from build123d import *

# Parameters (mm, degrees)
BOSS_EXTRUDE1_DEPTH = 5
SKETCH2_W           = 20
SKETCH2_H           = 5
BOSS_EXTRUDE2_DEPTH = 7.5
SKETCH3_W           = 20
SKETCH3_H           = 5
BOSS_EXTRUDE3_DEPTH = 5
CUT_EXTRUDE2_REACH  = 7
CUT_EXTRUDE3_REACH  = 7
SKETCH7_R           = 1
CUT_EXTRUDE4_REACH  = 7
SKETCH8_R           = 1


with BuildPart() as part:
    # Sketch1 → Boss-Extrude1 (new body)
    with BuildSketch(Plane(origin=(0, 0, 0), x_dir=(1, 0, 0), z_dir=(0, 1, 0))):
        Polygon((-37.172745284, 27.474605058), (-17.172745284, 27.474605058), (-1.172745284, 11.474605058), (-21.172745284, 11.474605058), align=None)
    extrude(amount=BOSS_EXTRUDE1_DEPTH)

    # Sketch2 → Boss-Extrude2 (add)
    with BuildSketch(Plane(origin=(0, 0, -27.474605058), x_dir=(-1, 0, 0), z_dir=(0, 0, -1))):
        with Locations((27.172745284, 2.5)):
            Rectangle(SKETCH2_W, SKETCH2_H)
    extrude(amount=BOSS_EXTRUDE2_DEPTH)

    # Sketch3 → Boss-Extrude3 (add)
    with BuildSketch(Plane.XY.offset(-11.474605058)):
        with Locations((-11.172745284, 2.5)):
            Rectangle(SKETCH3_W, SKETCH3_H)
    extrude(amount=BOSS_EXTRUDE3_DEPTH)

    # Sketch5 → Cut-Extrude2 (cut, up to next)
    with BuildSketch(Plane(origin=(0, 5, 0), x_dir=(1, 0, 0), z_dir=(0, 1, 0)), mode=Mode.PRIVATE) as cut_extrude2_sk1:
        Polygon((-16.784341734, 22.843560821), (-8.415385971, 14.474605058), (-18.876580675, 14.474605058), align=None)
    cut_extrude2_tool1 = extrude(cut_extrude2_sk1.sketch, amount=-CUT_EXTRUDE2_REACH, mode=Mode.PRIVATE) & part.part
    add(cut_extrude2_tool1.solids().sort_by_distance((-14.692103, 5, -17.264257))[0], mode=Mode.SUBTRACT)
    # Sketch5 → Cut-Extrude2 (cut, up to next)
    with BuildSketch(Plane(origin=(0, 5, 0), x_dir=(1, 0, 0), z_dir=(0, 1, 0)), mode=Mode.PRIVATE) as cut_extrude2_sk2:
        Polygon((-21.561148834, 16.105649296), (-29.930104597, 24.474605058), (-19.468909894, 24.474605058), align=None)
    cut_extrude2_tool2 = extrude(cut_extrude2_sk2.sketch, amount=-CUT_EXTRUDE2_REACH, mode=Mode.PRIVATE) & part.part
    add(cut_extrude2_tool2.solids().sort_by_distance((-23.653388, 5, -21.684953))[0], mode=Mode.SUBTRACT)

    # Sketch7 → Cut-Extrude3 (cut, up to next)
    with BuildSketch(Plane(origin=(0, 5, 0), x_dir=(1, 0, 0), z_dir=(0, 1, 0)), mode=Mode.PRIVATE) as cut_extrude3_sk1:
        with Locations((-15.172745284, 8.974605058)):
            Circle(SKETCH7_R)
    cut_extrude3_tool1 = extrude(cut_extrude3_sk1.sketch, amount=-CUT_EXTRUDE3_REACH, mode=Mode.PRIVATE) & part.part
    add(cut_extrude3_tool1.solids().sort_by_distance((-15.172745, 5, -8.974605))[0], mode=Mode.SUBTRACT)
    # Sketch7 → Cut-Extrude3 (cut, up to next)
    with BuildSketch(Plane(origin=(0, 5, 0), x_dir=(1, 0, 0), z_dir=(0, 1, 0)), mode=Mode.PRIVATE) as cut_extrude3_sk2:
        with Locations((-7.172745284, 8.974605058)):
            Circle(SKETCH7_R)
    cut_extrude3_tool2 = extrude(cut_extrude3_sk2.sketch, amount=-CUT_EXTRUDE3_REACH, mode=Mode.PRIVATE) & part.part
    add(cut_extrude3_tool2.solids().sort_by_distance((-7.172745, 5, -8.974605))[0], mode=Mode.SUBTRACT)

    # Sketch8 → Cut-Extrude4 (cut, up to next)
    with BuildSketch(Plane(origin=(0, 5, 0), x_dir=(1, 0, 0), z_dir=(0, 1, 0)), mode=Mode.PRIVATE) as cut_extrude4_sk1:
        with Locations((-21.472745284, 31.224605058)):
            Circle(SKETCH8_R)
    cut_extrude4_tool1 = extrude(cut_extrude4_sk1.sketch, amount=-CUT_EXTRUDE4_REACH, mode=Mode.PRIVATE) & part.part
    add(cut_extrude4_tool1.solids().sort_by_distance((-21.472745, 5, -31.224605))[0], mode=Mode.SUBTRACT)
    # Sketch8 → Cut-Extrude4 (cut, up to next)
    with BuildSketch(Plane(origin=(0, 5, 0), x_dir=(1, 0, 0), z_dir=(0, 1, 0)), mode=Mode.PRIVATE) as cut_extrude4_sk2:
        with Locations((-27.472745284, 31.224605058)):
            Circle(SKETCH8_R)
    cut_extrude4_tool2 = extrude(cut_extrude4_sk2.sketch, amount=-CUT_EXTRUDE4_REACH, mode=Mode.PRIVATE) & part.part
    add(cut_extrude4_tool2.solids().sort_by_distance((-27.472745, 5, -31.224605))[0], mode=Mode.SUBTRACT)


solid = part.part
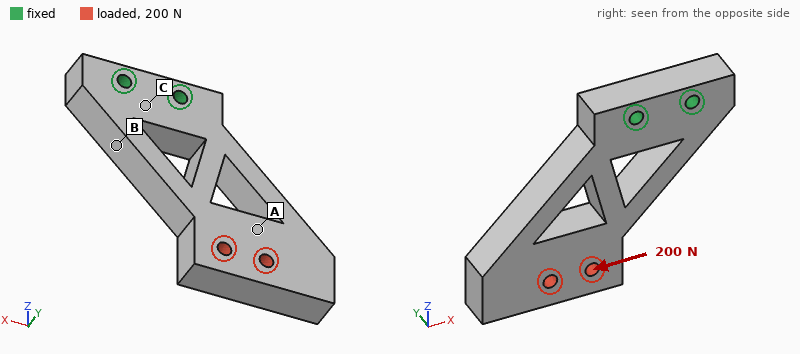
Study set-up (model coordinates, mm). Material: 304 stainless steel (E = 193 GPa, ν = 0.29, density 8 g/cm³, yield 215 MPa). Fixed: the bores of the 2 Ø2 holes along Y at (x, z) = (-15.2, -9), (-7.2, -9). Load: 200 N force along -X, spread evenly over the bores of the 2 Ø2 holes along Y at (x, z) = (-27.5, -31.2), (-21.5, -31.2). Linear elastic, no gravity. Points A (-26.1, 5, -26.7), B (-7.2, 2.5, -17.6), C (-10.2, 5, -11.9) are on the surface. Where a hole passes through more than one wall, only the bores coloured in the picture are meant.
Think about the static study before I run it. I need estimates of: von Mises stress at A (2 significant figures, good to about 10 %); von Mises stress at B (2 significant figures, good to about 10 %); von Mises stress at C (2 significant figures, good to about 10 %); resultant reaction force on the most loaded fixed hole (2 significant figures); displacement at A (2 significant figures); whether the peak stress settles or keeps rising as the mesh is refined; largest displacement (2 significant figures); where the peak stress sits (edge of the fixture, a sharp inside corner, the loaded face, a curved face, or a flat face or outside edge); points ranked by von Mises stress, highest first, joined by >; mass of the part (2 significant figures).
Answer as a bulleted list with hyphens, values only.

- 6.3 MPa
- 22 MPa
- 16 MPa
- 470 N
- 7.2 µm
- keeps rising
- 12 µm
- edge of the fixture
- B > C > A
- 19 g
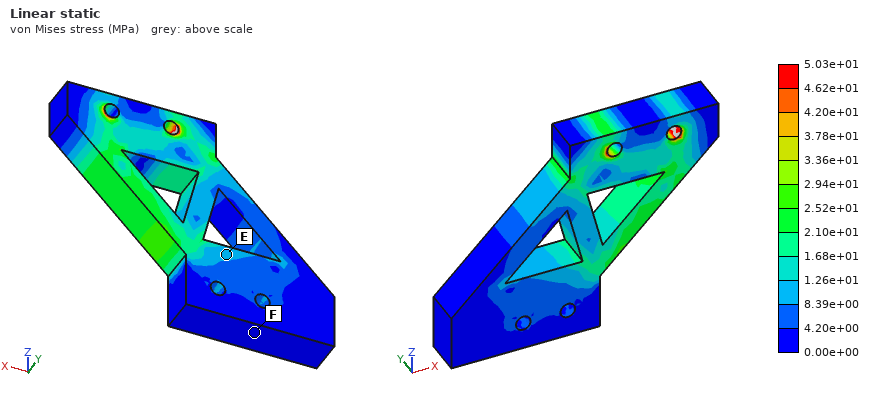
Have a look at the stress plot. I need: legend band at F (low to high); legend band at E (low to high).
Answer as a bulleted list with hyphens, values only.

- 0.00e+00 to 4.20e+00 MPa
- 8.39e+00 to 1.26e+01 MPa
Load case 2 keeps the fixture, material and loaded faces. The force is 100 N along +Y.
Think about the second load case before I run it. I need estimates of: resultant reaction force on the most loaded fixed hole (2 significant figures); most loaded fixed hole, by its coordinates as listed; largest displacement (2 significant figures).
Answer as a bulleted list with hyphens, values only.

- 120 N
- (-15.2, -9)
- 48 µm
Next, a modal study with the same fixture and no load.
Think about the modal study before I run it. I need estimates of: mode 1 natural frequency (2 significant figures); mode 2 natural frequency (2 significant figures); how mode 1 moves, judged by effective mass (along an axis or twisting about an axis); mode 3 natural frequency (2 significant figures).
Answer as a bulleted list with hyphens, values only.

- 3000 Hz
- 7200 Hz
- along Y
- 9200 Hz
